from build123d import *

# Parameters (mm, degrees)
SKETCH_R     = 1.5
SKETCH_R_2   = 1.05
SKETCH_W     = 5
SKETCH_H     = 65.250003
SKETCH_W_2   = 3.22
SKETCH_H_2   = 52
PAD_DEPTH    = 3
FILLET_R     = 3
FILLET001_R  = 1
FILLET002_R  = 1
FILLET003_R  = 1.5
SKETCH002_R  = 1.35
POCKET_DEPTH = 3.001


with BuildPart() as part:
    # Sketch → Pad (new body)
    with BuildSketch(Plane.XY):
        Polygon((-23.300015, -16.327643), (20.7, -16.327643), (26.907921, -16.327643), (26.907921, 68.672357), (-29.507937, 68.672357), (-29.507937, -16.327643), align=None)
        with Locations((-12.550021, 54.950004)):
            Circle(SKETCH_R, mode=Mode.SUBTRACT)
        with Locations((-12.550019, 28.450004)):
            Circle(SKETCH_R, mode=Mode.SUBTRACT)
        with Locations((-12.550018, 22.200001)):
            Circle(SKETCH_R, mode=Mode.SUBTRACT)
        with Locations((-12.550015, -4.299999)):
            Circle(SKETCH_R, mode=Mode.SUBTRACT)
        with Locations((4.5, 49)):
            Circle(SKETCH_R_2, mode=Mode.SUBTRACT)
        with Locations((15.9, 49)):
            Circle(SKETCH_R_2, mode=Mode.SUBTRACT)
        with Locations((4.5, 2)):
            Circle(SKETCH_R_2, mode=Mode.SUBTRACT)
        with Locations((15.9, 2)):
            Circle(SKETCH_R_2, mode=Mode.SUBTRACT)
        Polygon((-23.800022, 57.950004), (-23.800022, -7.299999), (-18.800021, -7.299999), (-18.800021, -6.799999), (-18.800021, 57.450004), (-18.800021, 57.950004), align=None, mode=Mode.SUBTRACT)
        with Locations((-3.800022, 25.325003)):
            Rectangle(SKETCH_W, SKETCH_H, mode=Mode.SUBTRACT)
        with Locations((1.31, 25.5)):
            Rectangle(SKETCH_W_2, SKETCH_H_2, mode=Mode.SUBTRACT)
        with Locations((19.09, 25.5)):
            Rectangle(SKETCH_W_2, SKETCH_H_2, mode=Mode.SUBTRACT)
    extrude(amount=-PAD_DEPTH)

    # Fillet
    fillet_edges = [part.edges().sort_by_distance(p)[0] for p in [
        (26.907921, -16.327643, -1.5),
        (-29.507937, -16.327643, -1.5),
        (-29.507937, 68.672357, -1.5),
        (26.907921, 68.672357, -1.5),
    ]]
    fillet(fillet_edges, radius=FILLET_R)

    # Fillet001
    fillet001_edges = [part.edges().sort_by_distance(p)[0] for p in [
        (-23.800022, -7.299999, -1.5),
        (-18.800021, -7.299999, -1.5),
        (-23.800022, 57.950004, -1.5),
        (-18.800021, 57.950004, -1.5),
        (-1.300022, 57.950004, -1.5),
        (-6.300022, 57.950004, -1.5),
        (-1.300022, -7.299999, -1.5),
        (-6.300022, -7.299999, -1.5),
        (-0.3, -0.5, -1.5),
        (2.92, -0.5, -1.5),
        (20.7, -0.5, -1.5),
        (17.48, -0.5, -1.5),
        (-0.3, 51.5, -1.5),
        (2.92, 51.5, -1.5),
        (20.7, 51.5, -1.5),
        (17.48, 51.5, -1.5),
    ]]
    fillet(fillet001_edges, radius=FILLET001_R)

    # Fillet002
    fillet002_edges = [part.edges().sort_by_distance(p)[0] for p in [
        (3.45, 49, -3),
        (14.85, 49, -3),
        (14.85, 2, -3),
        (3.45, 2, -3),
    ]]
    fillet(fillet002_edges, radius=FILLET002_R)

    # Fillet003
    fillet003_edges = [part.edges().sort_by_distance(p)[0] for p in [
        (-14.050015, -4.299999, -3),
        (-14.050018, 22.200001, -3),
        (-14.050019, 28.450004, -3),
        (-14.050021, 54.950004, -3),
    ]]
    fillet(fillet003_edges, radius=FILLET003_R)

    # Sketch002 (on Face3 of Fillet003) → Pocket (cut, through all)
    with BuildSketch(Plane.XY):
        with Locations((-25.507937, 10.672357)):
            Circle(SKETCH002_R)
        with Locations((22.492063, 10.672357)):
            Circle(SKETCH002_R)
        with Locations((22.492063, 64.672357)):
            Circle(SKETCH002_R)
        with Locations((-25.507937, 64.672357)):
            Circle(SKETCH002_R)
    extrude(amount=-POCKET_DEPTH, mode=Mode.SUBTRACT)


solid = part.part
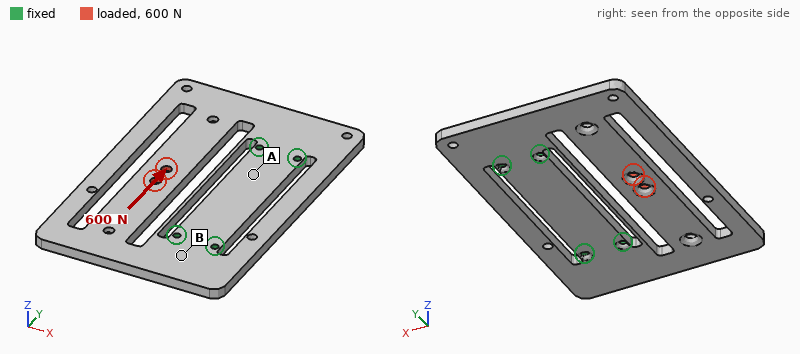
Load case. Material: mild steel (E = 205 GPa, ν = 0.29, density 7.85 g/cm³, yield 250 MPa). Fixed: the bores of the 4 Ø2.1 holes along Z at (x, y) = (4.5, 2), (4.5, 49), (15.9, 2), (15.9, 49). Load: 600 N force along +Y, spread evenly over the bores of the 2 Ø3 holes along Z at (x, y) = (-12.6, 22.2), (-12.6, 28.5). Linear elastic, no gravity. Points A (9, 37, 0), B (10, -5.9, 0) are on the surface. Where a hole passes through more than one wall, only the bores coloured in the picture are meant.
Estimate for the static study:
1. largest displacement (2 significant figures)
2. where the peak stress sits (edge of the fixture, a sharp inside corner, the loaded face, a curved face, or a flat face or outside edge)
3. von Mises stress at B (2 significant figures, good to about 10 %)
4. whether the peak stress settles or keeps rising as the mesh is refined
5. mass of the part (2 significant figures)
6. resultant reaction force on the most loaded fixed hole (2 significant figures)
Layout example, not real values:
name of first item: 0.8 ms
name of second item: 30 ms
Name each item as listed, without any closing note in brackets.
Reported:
largest displacement: 14 µm
where the peak stress sits: edge of the fixture
von Mises stress at B: 13 MPa
whether the peak stress settles or keeps rising as the mesh is refined: keeps rising
mass of the part: 88 g
resultant reaction force on the most loaded fixed hole: 590 N
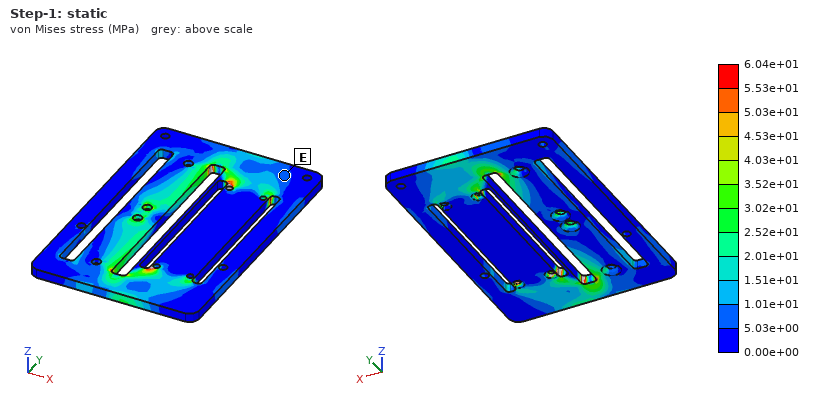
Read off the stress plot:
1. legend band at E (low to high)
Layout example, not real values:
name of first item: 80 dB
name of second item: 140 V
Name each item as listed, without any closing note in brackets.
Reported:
legend band at E: 5.03e+00 to 1.01e+01 MPa
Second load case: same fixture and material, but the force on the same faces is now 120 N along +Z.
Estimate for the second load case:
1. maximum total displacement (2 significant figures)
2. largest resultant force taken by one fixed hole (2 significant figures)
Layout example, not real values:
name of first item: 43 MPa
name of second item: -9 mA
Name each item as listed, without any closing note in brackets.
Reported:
maximum total displacement: 0.13 mm
largest resultant force taken by one fixed hole: 140 N
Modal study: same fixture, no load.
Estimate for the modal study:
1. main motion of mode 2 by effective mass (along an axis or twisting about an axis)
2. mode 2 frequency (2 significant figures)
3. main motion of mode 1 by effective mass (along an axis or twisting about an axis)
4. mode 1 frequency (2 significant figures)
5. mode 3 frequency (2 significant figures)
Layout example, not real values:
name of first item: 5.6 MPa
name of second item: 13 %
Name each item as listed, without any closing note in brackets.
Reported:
main motion of mode 2 by effective mass: twisting about X
mode 2 frequency: 1800 Hz
main motion of mode 1 by effective mass: along Z
mode 1 frequency: 910 Hz
mode 3 frequency: 1900 Hz
